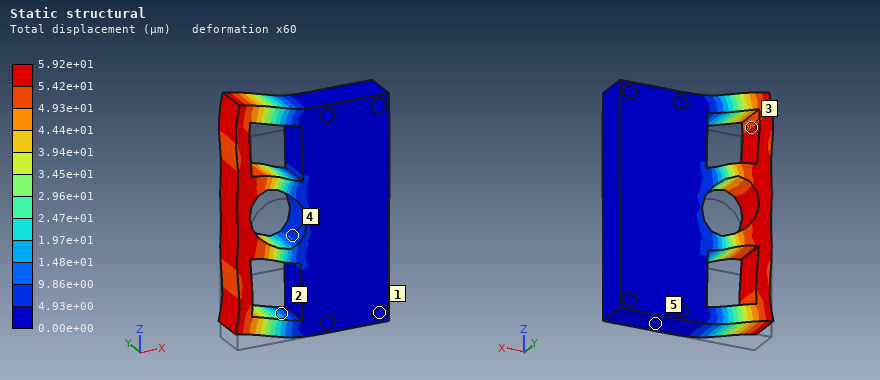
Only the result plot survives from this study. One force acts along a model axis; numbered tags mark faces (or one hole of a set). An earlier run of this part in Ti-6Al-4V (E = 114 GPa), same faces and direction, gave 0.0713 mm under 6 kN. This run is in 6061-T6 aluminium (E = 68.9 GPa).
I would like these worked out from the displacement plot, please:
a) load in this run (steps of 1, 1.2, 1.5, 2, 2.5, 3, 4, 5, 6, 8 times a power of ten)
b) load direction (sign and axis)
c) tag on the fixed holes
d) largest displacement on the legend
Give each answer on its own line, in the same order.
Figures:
3 kN
+Z
1
5.92e+01 µm
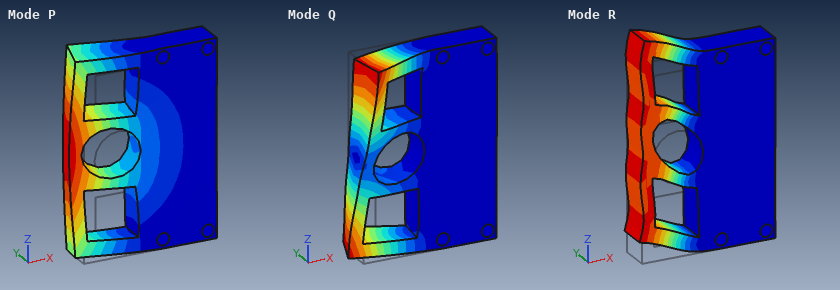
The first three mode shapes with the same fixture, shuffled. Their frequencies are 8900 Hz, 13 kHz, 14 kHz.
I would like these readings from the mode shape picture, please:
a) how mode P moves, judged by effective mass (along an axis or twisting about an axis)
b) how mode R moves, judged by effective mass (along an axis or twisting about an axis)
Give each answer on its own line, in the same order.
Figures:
along Y
along Z
